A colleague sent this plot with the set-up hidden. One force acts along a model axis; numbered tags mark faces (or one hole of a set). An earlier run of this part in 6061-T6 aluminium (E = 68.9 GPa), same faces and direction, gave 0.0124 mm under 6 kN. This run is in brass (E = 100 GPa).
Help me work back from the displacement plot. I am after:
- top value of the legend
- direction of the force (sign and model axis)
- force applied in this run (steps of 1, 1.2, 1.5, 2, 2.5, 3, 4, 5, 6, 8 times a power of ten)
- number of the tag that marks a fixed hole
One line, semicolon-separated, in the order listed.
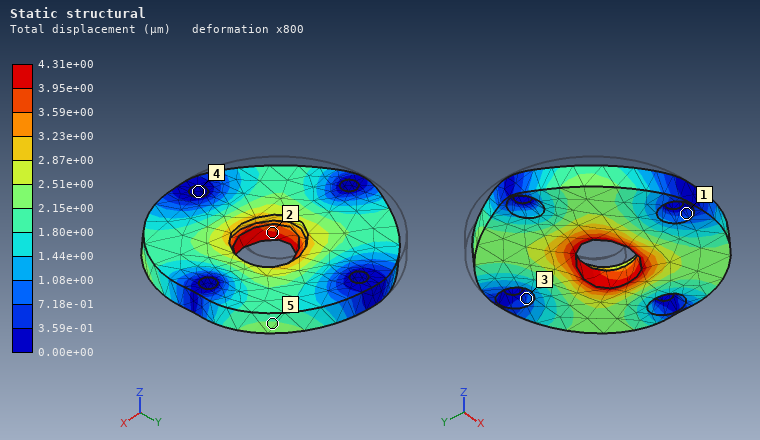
4.31e+00 µm; +X; 3 kN; 4
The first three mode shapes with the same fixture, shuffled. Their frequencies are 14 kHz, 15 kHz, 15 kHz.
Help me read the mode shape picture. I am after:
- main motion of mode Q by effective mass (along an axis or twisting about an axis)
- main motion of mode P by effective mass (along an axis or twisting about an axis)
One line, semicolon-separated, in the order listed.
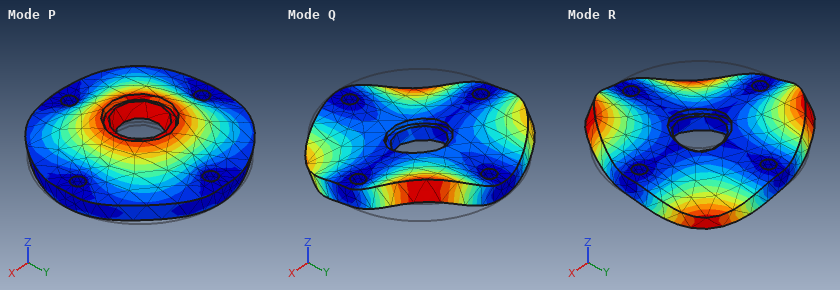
twisting about X; along Z
